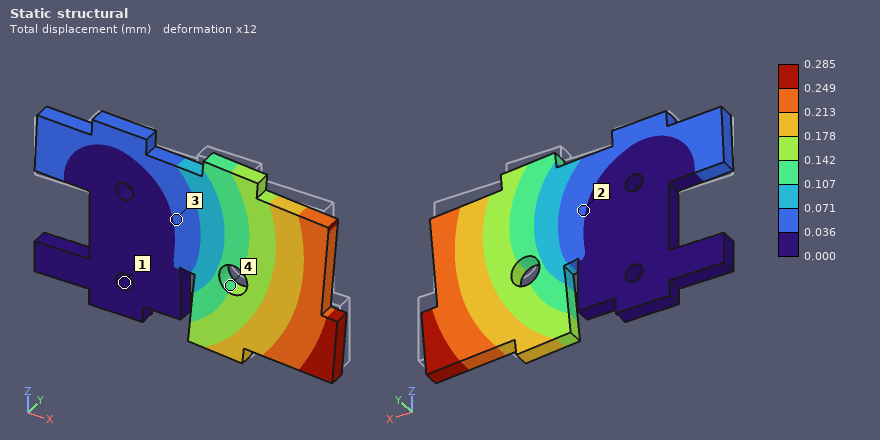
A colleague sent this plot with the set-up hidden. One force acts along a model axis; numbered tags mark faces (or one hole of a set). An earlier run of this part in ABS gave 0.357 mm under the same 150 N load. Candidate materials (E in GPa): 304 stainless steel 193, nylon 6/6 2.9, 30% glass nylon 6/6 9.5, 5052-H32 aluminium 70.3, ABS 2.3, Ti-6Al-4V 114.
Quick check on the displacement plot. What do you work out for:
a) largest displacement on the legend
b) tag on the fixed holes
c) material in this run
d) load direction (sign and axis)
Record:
0.285 mm
1
nylon 6/6
-Z
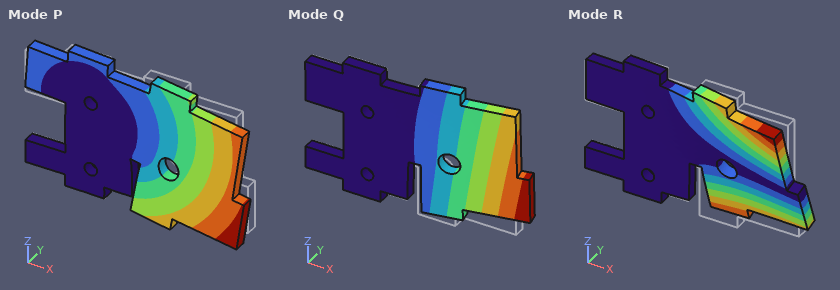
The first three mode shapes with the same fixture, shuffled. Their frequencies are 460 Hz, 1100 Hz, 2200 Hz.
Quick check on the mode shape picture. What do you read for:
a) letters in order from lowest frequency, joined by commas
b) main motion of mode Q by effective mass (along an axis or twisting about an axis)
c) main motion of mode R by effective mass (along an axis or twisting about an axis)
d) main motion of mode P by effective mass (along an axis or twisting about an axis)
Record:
Q, R, P
along Y
twisting about X
along Z
